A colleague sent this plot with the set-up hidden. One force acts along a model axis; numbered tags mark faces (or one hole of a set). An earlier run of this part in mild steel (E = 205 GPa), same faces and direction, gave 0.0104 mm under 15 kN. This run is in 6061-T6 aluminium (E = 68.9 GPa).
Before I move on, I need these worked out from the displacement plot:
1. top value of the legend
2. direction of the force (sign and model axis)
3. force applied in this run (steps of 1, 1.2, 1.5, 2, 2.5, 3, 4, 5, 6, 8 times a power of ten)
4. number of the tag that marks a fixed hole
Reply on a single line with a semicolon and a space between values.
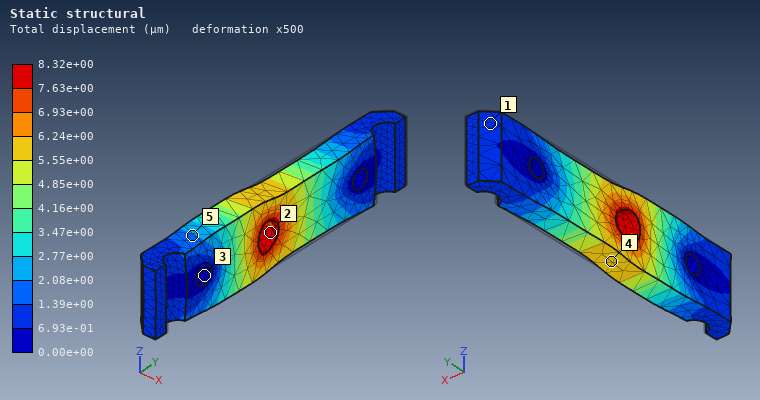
8.32e+00 µm; -Y; 4 kN; 3
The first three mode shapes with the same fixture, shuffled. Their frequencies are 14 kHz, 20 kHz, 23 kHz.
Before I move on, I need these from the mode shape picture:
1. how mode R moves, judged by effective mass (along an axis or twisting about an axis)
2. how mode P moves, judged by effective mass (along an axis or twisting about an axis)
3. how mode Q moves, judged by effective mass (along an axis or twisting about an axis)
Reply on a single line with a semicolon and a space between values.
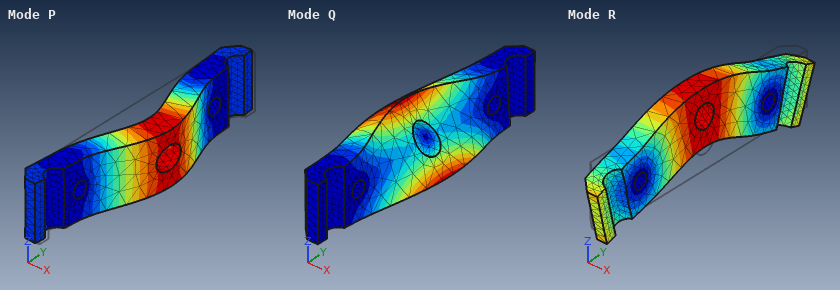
along Z; along X; twisting about Y
